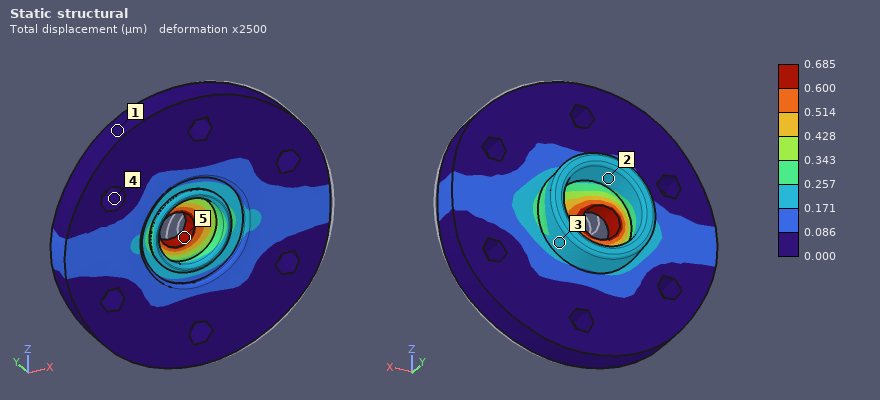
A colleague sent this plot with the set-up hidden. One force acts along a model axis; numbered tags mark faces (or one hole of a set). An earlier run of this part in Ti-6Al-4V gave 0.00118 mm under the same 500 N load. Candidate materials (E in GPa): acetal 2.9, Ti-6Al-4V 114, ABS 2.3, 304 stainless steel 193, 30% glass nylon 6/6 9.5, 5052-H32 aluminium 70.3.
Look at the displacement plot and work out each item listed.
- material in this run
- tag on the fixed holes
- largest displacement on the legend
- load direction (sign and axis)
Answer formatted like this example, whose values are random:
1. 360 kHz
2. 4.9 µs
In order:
1. 304 stainless steel
2. 4
3. 0.685 µm
4. -X
